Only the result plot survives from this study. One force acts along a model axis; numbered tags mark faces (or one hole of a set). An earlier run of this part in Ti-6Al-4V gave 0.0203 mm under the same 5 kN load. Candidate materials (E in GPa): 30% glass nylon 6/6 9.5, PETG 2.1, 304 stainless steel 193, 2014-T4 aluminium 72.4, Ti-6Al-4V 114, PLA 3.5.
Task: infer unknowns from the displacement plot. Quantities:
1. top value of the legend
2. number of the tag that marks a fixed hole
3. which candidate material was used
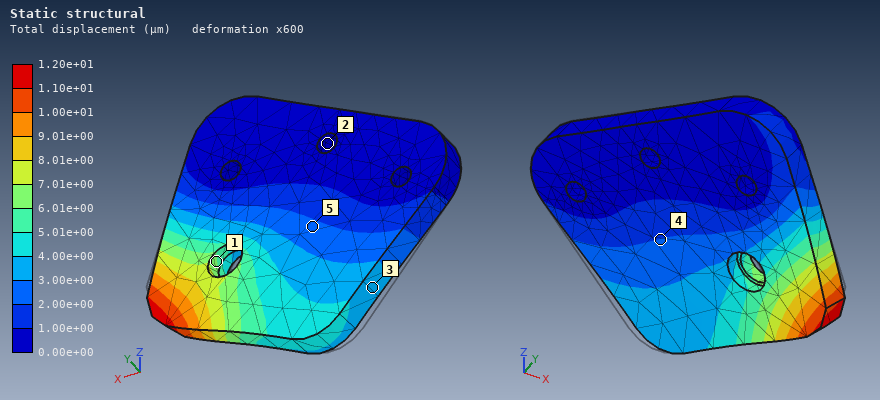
1.20e+01 µm
2
304 stainless steel
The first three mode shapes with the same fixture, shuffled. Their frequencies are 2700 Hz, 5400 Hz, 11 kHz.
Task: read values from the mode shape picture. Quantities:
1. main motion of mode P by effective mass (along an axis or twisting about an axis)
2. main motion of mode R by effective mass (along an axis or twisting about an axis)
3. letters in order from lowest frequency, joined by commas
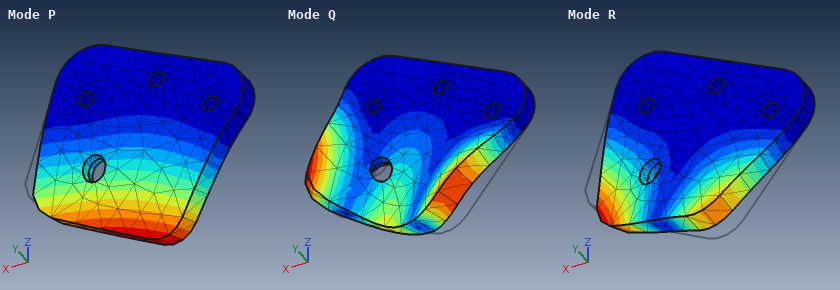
along Y
twisting about Z
P, R, Q
